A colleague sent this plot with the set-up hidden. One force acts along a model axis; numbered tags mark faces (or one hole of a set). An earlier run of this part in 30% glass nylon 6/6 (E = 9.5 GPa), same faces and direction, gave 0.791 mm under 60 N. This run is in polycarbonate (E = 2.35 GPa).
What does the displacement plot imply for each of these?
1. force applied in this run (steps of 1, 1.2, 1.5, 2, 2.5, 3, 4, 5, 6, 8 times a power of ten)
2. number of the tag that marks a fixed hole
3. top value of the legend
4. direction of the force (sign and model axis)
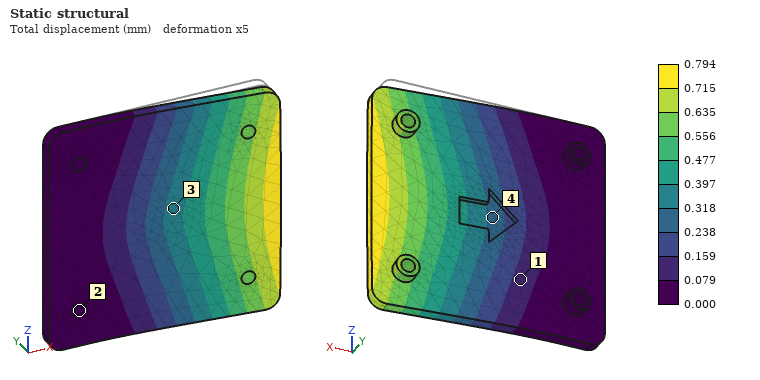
15 N
2
0.794 mm
-Y
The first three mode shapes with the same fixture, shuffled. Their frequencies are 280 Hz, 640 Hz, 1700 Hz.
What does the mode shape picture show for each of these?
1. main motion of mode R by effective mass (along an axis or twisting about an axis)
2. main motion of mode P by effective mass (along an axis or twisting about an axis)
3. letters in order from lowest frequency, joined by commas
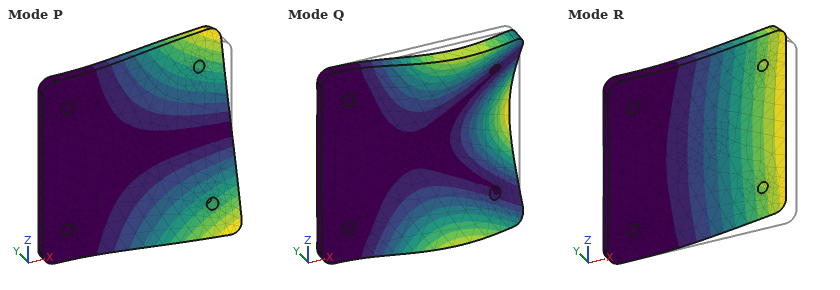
along Y
twisting about X
R, P, Q
